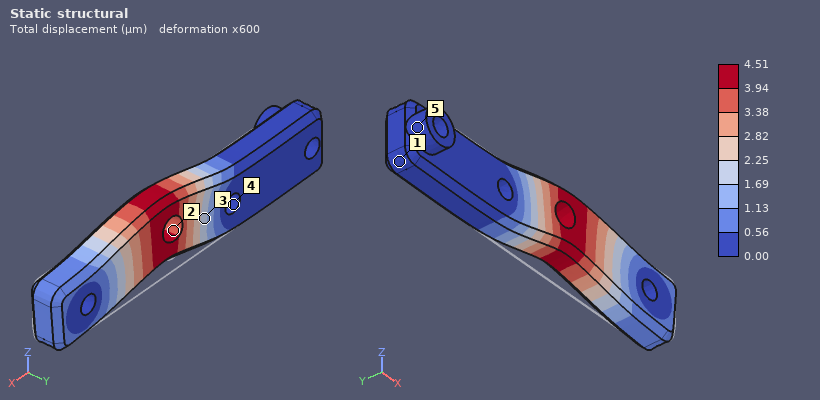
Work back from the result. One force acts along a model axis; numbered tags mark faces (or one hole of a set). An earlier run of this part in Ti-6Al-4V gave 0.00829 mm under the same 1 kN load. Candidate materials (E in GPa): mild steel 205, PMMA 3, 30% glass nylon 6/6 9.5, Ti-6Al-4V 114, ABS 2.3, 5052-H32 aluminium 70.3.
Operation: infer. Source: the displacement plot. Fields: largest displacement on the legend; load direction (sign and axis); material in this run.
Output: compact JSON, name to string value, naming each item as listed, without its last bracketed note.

{"largest displacement on the legend": "4.51 µm", "load direction": "+Z", "material in this run": "mild steel"}
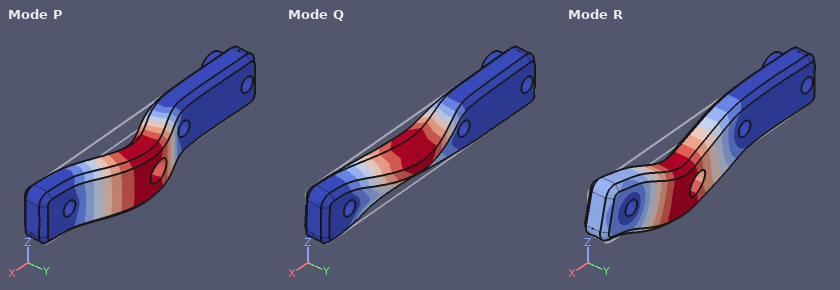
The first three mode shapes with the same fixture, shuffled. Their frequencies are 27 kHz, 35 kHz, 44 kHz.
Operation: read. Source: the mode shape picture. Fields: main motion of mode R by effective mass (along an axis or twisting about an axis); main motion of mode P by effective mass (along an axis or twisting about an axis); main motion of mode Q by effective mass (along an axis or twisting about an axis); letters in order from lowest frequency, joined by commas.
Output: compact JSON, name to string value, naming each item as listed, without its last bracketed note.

{"main motion of mode R by effective mass": "along Z", "main motion of mode P by effective mass": "along Y", "main motion of mode Q by effective mass": "twisting about X", "letters in order from lowest frequency, joined by commas": "P, R, Q"}
